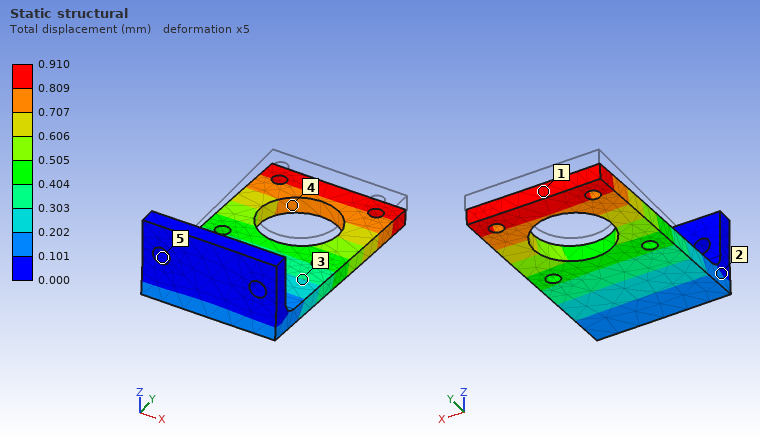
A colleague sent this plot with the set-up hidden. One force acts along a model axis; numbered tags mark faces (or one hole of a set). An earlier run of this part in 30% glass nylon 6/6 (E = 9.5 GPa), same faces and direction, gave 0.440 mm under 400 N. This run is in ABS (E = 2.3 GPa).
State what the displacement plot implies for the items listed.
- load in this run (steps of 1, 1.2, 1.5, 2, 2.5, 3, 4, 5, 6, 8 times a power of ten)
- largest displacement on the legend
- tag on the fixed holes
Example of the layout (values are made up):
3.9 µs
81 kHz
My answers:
200 N
0.910 mm
5
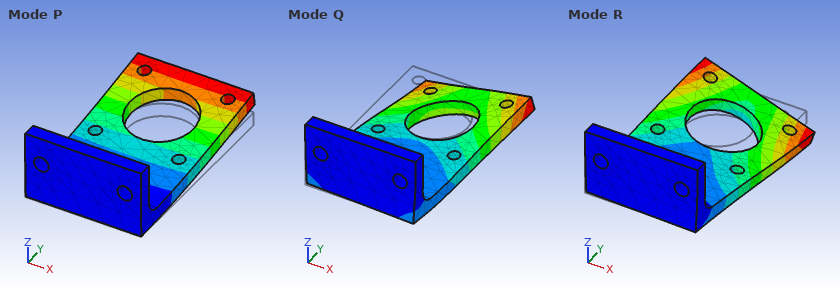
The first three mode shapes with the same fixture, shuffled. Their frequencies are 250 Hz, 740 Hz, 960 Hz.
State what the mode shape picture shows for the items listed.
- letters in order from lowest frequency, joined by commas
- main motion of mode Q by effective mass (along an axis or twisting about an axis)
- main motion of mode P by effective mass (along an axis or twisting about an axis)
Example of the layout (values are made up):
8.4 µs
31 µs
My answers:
P, R, Q
along X
along Z
